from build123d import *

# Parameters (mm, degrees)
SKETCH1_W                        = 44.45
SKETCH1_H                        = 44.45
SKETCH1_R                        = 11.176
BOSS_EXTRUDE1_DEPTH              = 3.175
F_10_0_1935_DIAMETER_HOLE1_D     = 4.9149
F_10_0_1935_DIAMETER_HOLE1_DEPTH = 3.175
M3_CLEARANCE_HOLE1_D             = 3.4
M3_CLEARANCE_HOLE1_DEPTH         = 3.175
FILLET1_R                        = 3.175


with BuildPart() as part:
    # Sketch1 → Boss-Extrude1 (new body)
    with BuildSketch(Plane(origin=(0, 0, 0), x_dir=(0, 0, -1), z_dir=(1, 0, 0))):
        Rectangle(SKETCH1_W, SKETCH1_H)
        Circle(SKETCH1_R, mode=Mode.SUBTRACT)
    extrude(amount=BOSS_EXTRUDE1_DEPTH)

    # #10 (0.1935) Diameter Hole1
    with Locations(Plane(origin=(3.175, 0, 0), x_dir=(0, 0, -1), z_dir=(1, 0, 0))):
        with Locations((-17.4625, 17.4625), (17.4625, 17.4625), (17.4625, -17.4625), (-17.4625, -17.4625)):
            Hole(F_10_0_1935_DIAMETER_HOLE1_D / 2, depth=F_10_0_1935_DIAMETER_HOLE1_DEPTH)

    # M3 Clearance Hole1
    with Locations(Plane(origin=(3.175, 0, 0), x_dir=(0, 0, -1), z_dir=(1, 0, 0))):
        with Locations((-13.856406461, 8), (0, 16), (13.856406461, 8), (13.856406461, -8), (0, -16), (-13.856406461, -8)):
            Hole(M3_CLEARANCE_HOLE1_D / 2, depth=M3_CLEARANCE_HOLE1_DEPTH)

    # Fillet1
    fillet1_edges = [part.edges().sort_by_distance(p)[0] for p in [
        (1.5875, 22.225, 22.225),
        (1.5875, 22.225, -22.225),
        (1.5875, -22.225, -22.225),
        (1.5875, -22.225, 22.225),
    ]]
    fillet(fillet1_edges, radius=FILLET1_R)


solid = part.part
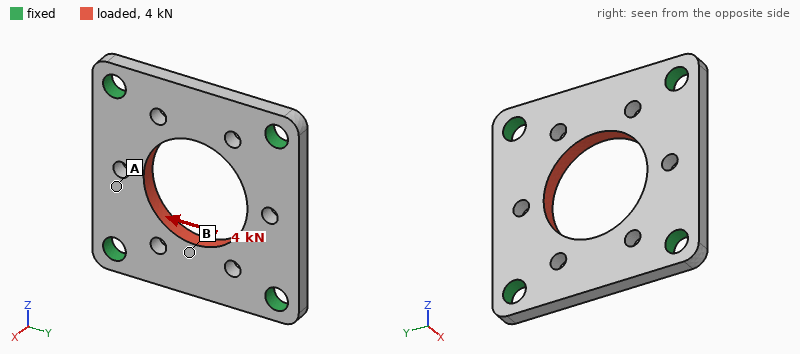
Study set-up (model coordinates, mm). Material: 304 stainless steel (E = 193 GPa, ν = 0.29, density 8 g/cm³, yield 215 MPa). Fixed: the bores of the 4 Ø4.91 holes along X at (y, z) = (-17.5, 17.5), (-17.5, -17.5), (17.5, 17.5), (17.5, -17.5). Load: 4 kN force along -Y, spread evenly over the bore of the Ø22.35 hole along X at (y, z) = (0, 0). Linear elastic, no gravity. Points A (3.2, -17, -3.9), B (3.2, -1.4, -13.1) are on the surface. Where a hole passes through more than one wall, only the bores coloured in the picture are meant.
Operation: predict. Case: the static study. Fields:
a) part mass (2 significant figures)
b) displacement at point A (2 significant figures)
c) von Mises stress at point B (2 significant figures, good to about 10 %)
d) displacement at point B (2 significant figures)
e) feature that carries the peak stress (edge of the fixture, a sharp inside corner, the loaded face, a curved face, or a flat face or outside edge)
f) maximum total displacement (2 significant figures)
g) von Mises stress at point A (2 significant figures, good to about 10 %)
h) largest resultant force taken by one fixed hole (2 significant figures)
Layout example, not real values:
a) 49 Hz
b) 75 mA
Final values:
a) 37 g
b) 3.5 µm
c) 31 MPa
d) 2.0 µm
e) edge of the fixture
f) 4.4 µm
g) 18 MPa
h) 1.1 kN
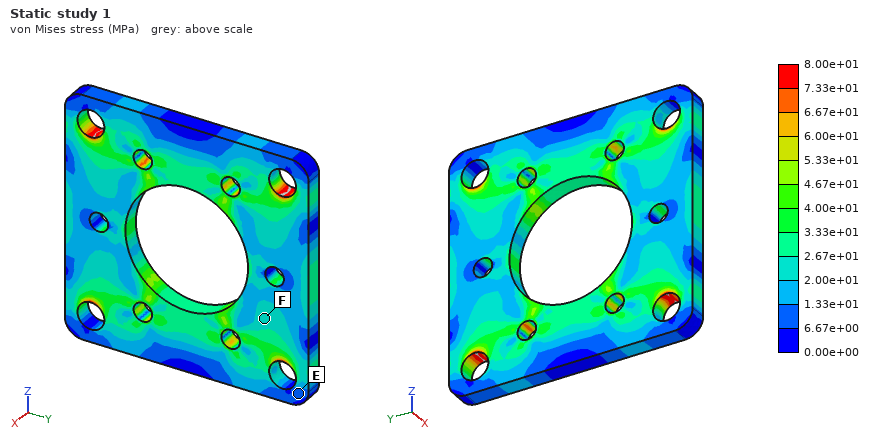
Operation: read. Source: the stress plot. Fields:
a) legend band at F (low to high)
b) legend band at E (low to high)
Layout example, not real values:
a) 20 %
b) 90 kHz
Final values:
a) 2.00e+01 to 2.67e+01 MPa
b) 6.67e+00 to 1.33e+01 MPa
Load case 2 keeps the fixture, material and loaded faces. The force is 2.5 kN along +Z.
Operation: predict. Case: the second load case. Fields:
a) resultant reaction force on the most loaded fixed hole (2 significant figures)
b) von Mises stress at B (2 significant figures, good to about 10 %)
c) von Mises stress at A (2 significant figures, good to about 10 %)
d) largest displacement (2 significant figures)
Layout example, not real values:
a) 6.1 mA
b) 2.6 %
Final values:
a) 650 N
b) 9.9 MPa
c) 13 MPa
d) 2.9 µm
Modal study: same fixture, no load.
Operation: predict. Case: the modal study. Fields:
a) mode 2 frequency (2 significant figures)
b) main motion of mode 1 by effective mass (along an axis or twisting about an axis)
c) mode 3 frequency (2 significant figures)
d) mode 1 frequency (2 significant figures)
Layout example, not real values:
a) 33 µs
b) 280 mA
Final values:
a) 15 kHz
b) along X
c) 16 kHz
d) 13 kHz
